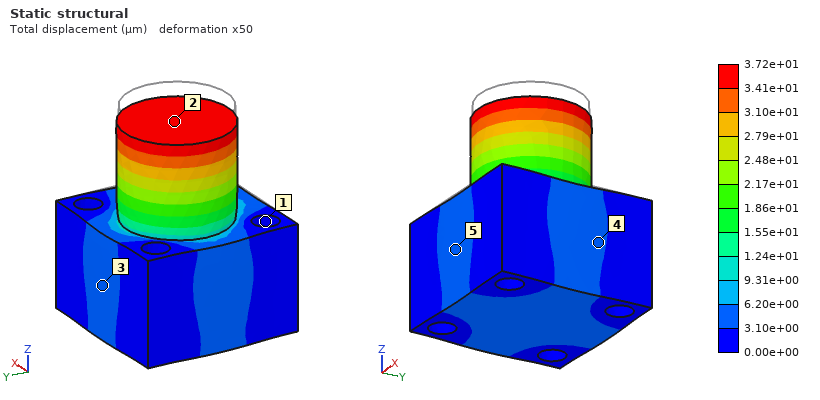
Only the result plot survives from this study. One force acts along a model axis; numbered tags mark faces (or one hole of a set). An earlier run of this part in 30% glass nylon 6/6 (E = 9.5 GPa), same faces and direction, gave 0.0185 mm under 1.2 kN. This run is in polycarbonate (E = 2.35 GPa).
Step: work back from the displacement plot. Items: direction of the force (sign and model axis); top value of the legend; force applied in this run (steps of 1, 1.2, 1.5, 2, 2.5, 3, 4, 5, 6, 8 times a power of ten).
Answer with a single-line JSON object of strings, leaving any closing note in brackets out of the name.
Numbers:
{"direction of the force": "-Z", "top value of the legend": "3.72e+01 µm", "force applied in this run": "600 N"}
